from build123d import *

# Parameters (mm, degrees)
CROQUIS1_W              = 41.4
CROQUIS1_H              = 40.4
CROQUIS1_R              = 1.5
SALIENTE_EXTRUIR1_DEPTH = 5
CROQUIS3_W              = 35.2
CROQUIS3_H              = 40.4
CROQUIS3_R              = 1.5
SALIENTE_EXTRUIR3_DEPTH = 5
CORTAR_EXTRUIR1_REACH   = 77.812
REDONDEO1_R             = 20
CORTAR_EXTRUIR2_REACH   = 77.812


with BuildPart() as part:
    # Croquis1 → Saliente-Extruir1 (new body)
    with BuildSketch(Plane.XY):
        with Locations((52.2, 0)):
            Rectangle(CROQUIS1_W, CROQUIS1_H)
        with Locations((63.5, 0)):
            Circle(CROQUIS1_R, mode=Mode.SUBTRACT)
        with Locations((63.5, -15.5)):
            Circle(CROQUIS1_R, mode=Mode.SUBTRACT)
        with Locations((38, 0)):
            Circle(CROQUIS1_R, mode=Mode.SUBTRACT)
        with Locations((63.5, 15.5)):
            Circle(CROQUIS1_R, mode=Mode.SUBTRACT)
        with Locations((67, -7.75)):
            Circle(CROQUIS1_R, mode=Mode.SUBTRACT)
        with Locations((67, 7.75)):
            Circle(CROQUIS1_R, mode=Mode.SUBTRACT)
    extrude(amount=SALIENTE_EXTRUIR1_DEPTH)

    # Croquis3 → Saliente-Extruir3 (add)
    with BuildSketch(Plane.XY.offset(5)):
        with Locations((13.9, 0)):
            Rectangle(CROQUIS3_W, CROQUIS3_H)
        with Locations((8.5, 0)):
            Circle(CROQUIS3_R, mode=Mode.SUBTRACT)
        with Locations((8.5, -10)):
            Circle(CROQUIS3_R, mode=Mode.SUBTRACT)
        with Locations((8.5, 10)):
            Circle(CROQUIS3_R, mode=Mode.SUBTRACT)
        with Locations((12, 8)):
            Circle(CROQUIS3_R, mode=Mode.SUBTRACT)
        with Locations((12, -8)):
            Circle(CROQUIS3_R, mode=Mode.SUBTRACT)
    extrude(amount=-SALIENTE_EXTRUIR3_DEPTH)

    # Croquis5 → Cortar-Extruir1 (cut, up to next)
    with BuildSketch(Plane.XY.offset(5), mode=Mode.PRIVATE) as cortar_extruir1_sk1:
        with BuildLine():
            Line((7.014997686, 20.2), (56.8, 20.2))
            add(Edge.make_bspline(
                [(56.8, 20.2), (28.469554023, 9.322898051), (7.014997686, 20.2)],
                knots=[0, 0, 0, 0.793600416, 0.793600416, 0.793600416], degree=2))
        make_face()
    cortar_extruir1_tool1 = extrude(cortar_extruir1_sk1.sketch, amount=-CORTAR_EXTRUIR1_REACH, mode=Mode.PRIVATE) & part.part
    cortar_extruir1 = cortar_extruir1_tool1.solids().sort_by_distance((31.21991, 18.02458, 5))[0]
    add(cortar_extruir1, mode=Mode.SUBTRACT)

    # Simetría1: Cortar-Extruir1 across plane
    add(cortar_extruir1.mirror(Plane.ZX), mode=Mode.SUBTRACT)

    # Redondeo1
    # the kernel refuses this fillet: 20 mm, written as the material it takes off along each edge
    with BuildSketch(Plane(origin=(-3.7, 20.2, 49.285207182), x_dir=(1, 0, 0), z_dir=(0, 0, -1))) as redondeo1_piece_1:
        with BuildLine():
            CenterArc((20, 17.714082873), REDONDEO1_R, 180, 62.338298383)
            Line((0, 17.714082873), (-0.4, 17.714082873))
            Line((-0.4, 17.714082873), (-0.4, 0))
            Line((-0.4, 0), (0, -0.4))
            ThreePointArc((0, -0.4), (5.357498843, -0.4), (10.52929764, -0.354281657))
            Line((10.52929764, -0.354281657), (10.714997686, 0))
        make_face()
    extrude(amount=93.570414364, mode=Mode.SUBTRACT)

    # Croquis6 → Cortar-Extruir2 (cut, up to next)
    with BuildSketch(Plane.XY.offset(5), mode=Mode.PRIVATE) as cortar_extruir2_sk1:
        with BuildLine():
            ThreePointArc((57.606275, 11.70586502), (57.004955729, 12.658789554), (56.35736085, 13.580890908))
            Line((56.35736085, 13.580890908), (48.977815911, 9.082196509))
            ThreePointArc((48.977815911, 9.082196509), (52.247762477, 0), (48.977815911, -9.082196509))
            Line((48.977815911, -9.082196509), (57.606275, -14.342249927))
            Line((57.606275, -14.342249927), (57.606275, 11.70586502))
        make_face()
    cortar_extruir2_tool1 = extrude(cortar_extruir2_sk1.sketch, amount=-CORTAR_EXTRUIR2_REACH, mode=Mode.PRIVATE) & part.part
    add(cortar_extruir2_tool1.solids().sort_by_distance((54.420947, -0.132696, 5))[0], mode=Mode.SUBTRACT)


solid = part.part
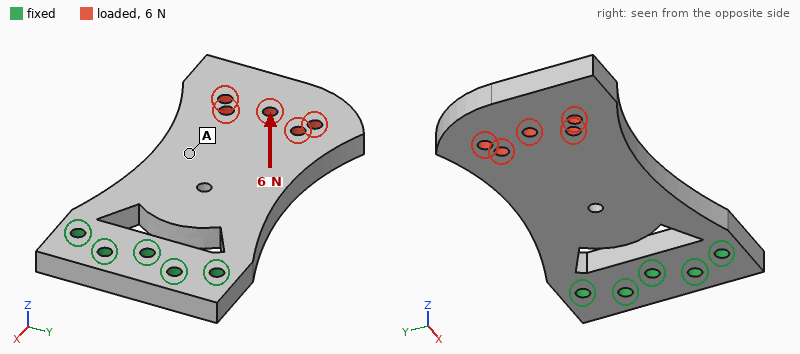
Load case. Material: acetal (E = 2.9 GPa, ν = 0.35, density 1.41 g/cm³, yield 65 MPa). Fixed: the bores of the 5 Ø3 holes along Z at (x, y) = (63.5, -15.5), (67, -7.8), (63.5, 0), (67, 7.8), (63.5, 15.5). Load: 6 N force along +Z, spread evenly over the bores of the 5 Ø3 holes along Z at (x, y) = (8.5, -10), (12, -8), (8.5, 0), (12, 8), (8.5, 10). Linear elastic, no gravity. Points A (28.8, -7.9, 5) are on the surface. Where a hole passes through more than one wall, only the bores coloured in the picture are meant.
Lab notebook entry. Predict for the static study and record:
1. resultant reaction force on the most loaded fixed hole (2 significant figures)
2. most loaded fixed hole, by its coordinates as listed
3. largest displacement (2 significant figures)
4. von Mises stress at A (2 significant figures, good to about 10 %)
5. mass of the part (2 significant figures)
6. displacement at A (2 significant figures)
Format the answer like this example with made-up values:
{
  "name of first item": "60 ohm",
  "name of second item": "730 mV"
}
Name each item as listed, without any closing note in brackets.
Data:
{
  "resultant reaction force on the most loaded fixed hole": "4.6 N",
  "most loaded fixed hole, by its coordinates as listed": "(63.5, 15.5)",
  "largest displacement": "0.82 mm",
  "von Mises stress at A": "0.95 MPa",
  "mass of the part": "17 g",
  "displacement at A": "0.33 mm"
}
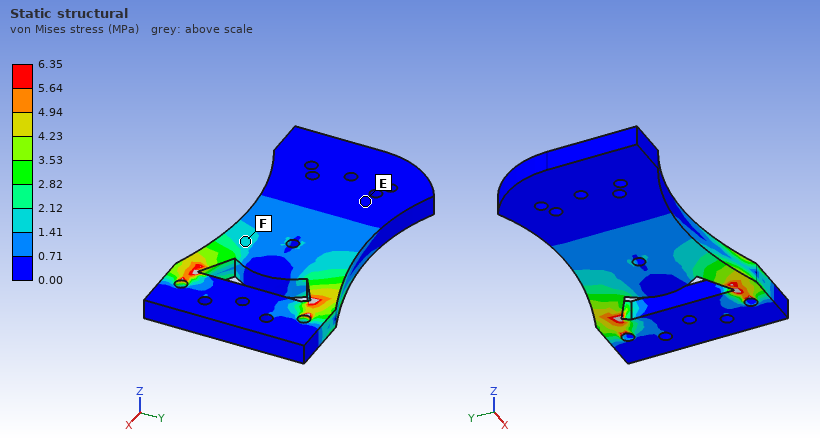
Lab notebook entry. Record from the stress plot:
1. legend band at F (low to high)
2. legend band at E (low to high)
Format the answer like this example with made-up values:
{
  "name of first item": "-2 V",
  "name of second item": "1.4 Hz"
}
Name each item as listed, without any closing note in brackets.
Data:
{
  "legend band at F": "1.41 to 2.12 MPa",
  "legend band at E": "0.00 to 0.71 MPa"
}
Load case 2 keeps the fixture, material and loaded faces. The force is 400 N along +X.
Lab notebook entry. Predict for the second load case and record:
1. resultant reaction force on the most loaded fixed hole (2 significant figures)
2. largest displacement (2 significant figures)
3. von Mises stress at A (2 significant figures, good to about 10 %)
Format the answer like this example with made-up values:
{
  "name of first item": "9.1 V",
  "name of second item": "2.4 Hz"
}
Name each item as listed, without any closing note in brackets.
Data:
{
  "resultant reaction force on the most loaded fixed hole": "220 N",
  "largest displacement": "90 µm",
  "von Mises stress at A": "2.6 MPa"
}
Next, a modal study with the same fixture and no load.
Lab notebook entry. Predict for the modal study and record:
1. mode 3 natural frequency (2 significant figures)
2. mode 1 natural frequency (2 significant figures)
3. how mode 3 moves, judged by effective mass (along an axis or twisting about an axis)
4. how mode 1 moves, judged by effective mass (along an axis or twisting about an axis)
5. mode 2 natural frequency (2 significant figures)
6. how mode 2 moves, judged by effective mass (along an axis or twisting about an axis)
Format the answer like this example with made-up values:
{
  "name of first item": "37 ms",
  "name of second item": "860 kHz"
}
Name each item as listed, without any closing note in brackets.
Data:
{
  "mode 3 natural frequency": "1400 Hz",
  "mode 1 natural frequency": "180 Hz",
  "how mode 3 moves, judged by effective mass": "along Y",
  "how mode 1 moves, judged by effective mass": "along Z",
  "mode 2 natural frequency": "930 Hz",
  "how mode 2 moves, judged by effective mass": "twisting about X"
}
